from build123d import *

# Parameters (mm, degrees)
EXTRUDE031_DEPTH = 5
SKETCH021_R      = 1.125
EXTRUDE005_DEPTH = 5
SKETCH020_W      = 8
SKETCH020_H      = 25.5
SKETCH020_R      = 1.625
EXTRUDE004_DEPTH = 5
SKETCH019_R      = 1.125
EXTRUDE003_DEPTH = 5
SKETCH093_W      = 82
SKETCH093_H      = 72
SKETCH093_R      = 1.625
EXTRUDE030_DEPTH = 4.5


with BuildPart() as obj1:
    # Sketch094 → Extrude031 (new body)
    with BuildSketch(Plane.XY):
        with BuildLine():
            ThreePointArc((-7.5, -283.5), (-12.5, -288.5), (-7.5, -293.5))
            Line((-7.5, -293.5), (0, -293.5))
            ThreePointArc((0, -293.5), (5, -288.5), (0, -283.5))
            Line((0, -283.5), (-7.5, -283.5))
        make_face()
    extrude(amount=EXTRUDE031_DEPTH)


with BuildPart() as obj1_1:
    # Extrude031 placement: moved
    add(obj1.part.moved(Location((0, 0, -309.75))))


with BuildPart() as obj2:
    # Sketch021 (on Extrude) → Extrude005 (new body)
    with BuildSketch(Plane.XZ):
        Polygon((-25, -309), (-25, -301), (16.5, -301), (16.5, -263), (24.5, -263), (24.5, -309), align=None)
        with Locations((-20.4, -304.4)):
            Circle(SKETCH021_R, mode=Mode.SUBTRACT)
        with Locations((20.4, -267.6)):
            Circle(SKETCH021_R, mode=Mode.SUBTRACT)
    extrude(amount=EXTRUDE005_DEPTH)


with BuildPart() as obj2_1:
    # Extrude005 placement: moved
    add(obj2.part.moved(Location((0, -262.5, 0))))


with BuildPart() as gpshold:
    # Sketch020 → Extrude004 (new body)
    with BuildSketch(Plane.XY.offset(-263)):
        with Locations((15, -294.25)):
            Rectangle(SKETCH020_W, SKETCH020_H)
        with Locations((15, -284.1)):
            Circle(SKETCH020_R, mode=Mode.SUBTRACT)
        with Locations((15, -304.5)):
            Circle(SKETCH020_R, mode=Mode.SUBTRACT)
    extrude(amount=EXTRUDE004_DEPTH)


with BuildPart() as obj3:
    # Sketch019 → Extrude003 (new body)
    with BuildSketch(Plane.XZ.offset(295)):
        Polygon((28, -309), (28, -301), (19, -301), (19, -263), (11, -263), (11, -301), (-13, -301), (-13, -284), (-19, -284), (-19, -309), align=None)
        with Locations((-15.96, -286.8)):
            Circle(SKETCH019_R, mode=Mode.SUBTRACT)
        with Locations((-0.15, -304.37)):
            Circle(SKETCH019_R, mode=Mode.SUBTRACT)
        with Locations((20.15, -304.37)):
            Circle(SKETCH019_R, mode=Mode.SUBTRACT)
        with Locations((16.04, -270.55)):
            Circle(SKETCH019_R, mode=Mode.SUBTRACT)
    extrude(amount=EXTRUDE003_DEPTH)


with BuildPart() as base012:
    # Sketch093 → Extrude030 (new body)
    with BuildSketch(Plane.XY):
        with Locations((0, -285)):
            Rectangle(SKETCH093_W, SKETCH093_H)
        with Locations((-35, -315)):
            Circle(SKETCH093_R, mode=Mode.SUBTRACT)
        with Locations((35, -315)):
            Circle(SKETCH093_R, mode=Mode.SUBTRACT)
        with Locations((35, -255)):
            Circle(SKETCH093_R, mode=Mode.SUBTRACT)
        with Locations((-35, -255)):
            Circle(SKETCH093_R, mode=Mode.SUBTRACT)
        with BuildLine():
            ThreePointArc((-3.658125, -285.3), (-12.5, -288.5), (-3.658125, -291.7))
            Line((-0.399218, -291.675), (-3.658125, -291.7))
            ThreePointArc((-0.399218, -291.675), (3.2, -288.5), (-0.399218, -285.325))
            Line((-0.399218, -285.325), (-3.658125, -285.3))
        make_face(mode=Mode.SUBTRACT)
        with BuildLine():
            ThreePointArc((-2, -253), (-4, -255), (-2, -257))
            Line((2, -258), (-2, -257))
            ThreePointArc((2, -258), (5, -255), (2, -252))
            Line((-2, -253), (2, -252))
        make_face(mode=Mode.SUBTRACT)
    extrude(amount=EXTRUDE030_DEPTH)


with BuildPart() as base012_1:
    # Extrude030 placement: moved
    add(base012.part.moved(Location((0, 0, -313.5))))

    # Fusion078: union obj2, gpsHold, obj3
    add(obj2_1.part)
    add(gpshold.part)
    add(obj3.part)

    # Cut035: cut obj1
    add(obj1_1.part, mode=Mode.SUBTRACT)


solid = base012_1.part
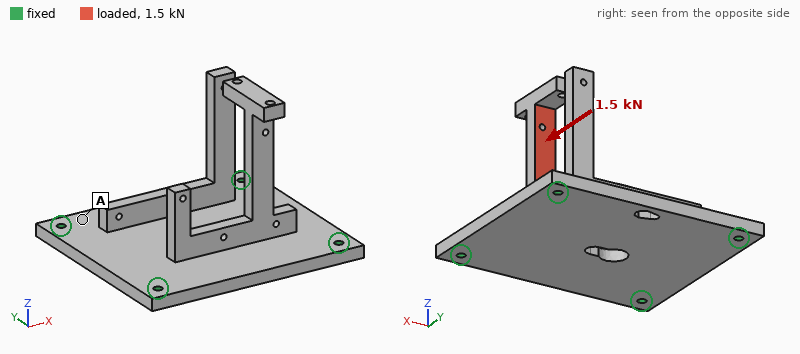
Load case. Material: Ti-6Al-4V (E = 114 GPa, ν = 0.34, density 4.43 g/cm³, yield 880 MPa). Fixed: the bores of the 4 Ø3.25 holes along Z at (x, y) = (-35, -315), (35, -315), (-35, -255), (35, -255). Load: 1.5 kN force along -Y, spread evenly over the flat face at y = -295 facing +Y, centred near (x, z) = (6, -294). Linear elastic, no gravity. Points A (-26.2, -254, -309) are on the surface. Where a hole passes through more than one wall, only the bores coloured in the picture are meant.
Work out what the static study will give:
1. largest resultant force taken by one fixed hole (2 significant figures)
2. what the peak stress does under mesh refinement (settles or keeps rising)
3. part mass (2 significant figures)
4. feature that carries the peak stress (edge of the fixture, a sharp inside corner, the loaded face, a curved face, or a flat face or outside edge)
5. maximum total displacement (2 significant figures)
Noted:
620 N
keeps rising
150 g
a sharp inside corner
1.1 mm
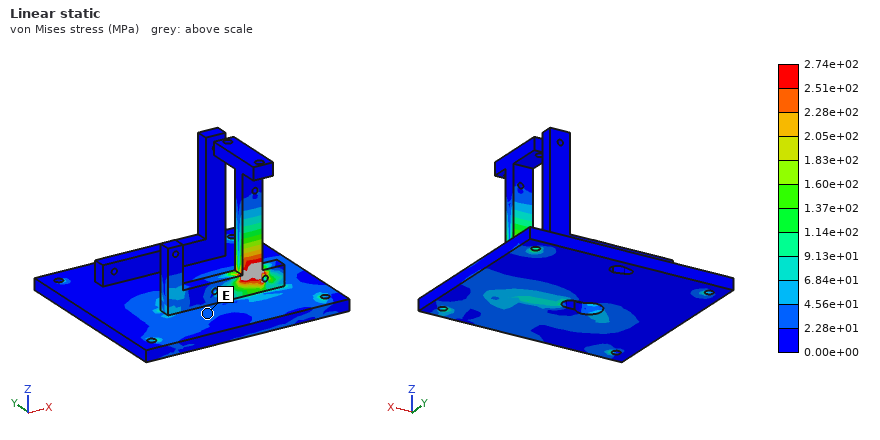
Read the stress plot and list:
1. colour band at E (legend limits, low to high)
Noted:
2.28e+01 to 4.56e+01 MPa
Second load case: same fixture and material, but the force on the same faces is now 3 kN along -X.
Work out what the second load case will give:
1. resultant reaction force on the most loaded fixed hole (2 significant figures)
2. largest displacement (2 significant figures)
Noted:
1.3 kN
0.76 mm
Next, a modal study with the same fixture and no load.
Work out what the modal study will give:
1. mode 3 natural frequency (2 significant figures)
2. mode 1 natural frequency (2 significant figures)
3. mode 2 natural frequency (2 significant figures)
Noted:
1900 Hz
1100 Hz
1800 Hz
